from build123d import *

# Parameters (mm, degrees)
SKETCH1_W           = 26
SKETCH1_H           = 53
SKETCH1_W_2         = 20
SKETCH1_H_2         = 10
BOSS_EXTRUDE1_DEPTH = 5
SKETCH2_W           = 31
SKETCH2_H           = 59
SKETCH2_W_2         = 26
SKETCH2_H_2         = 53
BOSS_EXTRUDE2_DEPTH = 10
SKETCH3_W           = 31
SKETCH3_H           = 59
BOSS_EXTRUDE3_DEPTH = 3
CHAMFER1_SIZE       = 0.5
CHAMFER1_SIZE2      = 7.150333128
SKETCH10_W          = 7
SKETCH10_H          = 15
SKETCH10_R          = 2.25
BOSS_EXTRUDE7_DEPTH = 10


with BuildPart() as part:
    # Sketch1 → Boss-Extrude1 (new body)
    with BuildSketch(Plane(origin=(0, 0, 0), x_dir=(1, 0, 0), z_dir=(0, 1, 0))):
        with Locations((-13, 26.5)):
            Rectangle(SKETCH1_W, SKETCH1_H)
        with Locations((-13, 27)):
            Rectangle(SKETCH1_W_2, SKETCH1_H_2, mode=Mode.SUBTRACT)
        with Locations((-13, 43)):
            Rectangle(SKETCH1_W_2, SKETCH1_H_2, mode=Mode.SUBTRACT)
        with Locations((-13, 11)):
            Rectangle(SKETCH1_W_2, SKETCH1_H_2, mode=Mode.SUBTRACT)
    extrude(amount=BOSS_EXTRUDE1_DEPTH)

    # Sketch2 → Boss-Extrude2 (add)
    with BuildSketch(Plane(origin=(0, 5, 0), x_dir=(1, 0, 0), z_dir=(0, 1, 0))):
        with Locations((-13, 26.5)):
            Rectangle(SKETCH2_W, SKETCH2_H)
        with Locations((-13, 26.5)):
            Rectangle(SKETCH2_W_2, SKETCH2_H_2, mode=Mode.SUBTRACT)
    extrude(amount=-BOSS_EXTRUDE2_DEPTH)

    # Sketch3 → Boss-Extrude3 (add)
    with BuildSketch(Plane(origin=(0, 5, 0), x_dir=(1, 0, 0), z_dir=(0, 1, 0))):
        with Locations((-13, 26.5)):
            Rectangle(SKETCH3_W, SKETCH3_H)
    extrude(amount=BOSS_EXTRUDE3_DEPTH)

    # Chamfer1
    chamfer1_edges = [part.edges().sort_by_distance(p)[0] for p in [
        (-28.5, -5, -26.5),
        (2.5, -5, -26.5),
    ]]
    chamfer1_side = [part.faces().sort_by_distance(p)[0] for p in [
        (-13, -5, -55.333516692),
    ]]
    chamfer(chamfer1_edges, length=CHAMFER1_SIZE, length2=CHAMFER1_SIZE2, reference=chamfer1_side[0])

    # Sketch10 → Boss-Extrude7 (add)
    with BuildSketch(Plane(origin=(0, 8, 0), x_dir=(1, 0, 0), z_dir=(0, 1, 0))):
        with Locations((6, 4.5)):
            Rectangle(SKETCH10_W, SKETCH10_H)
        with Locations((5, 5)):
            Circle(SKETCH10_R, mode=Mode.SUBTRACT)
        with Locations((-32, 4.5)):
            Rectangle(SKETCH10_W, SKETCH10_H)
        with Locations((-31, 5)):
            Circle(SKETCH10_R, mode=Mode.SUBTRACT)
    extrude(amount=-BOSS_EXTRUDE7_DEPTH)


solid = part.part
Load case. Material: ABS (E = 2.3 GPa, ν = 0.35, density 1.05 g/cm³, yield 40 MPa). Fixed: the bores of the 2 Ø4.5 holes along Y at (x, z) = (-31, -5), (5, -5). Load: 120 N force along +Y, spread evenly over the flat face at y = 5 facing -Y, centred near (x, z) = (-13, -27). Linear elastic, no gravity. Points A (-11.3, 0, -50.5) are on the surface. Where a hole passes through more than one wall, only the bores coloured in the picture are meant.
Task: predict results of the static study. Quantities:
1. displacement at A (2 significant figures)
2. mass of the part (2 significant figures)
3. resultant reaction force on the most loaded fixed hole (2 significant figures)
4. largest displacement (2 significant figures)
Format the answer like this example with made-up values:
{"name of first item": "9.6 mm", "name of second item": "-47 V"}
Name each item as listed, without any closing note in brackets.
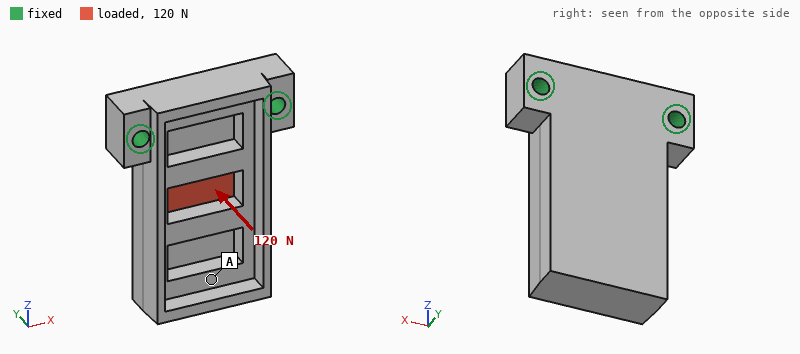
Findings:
{"displacement at A": "0.48 mm", "mass of the part": "16 g", "resultant reaction force on the most loaded fixed hole": "60 N", "largest displacement": "0.55 mm"}
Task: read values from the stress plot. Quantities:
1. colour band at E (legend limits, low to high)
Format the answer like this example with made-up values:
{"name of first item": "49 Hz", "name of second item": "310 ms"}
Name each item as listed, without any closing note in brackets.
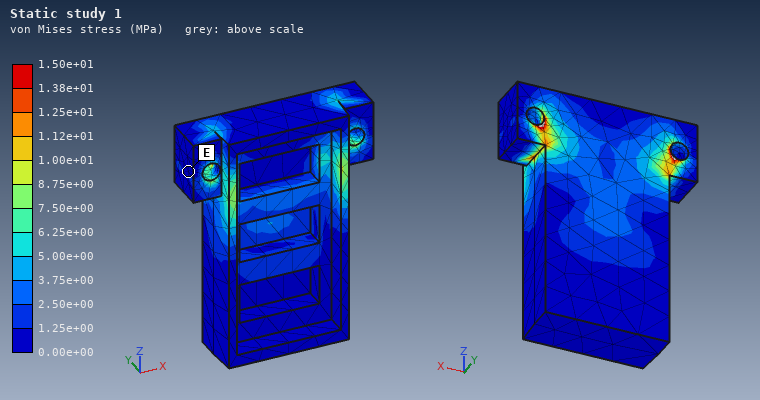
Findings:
{"colour band at E": "0.00e+00 to 1.25e+00 MPa"}
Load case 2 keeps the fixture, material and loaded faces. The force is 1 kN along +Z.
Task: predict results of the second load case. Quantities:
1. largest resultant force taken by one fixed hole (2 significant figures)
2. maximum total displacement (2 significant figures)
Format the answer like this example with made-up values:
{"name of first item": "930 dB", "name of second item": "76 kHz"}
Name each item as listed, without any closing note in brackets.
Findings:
{"largest resultant force taken by one fixed hole": "510 N", "maximum total displacement": "0.26 mm"}
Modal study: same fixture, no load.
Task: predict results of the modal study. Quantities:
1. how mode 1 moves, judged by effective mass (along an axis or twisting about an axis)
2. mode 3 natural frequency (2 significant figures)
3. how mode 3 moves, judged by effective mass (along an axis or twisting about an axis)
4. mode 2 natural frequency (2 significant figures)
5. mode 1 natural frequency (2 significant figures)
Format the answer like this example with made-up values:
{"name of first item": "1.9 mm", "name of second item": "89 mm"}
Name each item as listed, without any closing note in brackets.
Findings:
{"how mode 1 moves, judged by effective mass": "along Y", "mode 3 natural frequency": "2300 Hz", "how mode 3 moves, judged by effective mass": "along X", "mode 2 natural frequency": "1400 Hz", "mode 1 natural frequency": "670 Hz"}
